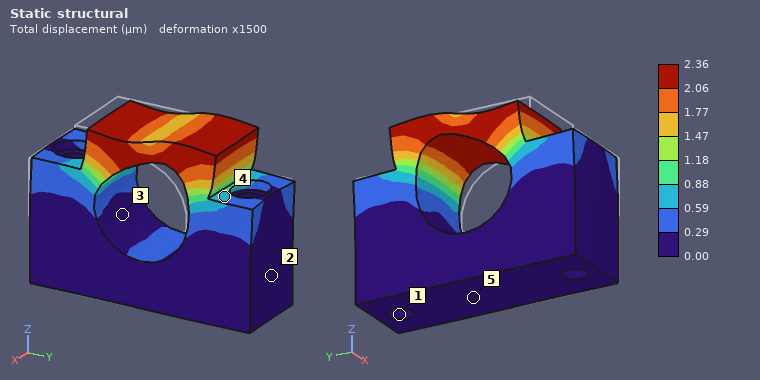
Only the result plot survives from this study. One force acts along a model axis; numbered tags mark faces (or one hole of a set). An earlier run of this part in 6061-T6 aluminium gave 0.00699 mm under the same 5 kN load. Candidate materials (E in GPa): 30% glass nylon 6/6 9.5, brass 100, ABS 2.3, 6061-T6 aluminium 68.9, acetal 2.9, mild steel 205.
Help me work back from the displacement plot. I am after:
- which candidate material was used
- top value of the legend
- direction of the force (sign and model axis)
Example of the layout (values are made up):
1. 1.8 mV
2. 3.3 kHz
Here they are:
1. mild steel
2. 2.36 µm
3. +Y
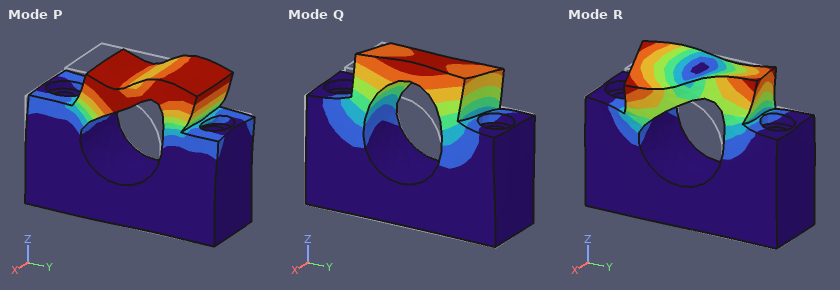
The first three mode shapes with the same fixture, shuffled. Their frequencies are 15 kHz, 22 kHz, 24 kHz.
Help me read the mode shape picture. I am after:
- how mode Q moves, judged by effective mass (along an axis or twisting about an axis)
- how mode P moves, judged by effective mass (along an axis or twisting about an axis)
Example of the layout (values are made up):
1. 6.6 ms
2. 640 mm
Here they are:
1. along X
2. along Y
